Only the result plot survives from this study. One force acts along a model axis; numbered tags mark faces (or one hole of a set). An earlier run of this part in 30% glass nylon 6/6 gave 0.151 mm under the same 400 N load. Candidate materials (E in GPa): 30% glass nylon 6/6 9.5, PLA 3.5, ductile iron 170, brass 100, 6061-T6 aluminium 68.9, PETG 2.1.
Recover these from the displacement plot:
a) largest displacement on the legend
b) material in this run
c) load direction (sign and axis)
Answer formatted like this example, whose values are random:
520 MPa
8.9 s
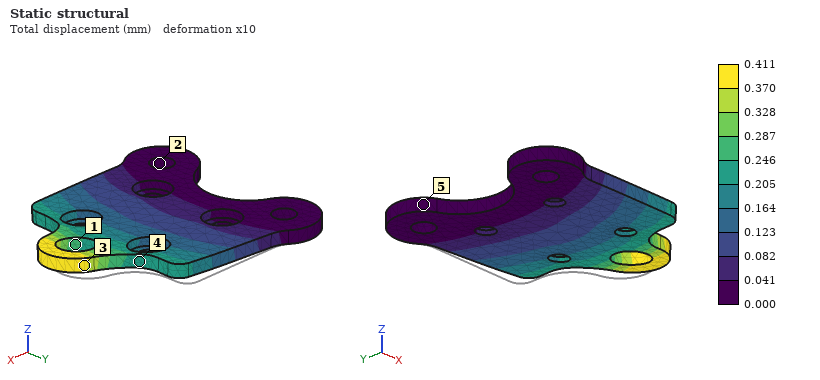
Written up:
0.411 mm
PLA
-Y
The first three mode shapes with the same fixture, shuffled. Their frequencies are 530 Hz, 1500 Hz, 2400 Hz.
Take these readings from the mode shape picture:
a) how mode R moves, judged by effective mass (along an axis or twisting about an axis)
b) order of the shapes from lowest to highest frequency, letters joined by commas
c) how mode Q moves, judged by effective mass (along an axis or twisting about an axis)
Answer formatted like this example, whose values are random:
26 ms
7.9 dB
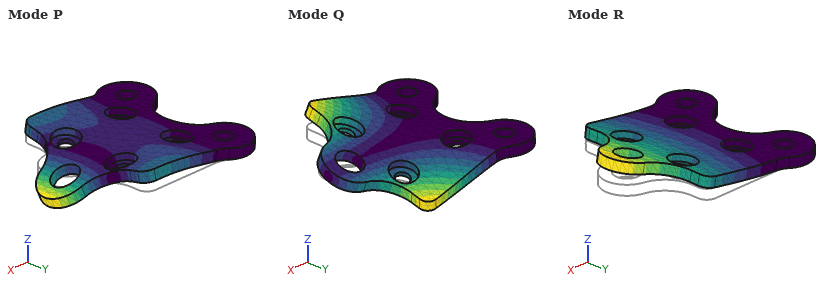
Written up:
along Z
R, Q, P
twisting about X
